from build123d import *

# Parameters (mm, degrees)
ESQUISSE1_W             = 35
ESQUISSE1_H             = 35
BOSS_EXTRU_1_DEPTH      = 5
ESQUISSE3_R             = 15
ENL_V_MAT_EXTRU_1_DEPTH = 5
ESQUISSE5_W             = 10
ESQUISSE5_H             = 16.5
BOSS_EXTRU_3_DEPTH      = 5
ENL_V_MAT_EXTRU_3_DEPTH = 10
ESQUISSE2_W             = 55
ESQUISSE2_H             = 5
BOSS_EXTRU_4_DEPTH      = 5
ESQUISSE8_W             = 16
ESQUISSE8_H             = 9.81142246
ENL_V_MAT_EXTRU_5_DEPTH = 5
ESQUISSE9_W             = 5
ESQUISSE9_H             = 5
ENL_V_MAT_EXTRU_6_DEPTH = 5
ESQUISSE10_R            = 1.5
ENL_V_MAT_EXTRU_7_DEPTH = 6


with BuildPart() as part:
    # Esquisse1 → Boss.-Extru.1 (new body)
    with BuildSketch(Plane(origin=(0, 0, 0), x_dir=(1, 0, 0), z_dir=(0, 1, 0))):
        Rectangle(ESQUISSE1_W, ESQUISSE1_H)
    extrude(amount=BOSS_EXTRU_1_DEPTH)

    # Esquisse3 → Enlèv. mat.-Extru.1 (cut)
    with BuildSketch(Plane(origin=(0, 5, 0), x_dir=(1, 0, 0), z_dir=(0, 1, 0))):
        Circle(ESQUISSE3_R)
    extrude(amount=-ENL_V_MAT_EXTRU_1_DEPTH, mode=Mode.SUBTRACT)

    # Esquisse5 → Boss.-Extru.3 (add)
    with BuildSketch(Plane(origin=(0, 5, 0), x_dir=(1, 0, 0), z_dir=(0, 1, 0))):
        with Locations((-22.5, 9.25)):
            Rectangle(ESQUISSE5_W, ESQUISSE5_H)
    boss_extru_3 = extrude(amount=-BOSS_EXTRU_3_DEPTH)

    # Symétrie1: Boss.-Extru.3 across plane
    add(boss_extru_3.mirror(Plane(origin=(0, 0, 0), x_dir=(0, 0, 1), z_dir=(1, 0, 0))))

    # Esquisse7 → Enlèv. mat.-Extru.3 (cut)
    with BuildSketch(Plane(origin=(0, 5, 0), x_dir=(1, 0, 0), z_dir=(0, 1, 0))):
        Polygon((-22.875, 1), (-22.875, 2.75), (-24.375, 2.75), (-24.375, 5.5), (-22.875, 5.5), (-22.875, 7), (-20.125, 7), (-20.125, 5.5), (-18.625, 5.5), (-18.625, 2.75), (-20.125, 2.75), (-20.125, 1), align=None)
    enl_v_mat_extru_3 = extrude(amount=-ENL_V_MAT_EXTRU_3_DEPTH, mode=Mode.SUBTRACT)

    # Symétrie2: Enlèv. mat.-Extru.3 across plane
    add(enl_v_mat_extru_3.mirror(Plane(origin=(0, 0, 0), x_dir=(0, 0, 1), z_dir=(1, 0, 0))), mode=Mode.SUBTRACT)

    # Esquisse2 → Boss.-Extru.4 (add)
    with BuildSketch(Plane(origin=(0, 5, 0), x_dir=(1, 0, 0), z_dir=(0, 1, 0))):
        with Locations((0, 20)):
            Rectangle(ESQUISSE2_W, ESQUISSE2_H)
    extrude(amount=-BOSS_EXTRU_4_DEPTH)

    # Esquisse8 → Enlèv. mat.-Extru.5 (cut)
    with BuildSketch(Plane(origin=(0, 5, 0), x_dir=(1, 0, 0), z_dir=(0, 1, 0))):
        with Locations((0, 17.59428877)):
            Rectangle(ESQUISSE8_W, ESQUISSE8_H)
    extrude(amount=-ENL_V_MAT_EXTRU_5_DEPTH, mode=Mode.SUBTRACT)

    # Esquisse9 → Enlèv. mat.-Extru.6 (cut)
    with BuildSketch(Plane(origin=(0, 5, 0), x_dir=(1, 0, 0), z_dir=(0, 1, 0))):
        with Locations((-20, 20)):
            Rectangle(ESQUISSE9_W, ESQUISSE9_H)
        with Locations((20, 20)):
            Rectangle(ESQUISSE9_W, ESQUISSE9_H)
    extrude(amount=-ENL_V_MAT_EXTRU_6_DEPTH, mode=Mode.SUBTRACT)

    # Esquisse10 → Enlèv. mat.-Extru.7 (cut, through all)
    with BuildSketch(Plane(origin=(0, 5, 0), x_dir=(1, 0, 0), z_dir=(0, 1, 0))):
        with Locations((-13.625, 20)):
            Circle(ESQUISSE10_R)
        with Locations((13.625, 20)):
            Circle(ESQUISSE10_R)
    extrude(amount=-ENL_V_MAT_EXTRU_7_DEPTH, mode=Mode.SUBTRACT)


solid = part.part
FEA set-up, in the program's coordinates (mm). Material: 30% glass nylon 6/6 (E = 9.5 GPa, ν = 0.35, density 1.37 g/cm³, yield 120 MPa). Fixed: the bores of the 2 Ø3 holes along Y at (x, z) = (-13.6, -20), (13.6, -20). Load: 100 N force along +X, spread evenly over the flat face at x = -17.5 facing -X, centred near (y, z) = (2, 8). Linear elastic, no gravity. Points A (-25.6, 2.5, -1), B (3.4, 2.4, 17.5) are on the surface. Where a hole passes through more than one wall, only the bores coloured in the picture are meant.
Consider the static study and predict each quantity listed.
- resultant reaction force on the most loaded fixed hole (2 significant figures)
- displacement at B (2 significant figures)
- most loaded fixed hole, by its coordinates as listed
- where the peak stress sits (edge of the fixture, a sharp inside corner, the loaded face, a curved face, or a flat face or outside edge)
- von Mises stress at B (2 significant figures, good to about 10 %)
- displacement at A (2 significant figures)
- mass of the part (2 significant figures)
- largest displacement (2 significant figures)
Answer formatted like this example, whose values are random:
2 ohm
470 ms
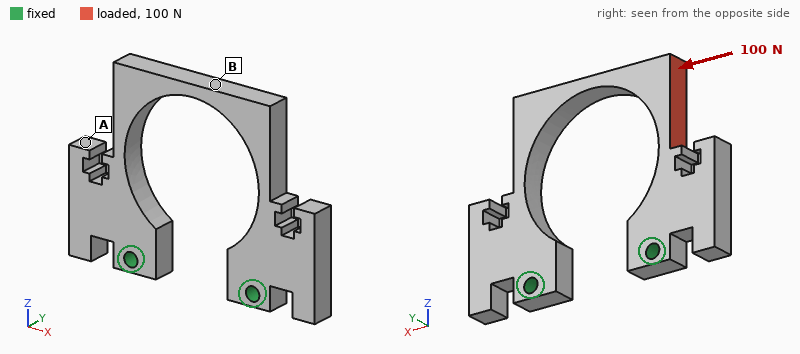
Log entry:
74 N
0.21 mm
(-13.6, -20)
edge of the fixture
15 MPa
0.12 mm
6.0 g
0.21 mm
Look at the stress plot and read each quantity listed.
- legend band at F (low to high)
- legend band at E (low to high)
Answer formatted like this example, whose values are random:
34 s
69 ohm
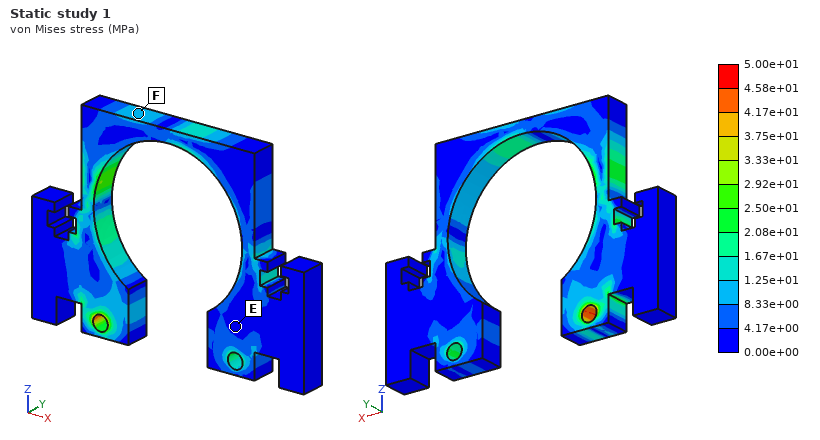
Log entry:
8.33e+00 to 1.25e+01 MPa
0.00e+00 to 4.17e+00 MPa
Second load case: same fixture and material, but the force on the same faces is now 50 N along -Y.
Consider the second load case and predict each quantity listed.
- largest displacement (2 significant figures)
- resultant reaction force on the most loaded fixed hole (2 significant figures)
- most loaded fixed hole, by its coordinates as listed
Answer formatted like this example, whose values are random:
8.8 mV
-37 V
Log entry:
0.67 mm
46 N
(-13.6, -20)
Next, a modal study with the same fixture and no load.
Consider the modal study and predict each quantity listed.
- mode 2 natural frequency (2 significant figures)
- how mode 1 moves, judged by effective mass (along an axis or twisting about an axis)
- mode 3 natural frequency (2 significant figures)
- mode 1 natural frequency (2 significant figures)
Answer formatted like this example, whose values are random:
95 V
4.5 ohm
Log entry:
2300 Hz
along Y
2400 Hz
1200 Hz
